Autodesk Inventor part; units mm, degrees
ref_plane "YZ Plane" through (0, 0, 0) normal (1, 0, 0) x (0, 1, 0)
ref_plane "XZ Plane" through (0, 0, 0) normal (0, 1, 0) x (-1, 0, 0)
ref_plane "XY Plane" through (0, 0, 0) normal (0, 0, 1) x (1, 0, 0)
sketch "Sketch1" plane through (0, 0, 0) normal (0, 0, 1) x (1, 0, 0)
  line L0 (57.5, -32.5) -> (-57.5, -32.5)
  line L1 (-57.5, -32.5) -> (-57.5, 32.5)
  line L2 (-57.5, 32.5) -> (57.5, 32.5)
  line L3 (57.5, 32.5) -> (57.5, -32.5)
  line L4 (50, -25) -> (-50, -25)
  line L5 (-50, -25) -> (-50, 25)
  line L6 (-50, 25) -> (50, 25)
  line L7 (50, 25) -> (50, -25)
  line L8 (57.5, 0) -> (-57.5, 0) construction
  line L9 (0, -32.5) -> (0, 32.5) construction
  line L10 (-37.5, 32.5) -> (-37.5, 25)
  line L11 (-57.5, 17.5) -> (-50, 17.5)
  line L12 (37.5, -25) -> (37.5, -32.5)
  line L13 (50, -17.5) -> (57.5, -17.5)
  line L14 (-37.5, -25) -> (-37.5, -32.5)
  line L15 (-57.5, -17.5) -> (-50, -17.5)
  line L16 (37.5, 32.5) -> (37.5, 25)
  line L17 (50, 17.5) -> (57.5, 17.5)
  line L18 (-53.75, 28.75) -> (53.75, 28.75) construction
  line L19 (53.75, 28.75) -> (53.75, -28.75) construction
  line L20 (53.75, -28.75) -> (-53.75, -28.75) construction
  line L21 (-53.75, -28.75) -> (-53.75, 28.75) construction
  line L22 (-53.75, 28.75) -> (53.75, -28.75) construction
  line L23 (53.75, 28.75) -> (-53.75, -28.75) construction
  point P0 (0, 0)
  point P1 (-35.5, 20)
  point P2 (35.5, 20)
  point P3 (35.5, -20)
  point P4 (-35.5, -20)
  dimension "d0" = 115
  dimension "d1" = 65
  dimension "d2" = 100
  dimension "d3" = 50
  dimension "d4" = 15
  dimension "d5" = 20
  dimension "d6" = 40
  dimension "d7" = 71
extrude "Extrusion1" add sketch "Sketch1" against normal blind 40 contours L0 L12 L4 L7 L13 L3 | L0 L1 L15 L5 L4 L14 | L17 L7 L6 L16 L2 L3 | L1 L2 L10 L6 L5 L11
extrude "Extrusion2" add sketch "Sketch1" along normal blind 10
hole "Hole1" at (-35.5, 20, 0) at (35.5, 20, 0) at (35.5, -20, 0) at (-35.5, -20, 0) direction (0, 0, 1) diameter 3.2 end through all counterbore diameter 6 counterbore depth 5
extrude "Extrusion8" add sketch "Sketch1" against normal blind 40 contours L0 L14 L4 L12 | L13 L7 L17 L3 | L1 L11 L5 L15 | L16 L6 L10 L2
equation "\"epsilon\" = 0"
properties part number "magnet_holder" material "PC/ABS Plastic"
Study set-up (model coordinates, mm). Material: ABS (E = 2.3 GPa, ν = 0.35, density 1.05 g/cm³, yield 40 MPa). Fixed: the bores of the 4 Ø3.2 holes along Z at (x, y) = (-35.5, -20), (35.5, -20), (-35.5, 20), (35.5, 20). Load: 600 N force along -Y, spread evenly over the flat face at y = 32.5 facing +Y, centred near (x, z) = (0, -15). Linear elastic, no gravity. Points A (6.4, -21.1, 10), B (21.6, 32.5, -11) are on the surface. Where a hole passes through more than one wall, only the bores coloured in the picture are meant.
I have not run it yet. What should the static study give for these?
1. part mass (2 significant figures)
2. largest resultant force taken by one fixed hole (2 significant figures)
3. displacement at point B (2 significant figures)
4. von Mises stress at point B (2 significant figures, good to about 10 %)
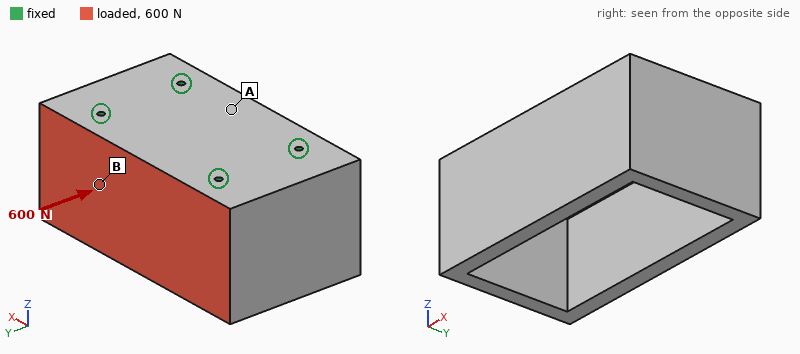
180 g
220 N
0.13 mm
2.1 MPa
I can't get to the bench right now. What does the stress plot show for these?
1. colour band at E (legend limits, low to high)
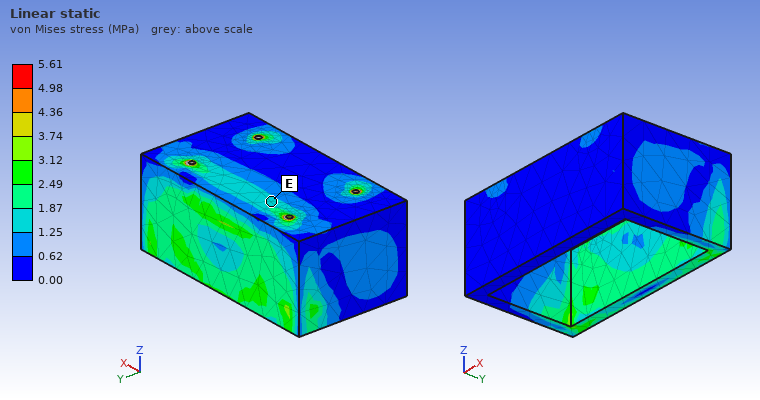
1.25 to 1.87 MPa
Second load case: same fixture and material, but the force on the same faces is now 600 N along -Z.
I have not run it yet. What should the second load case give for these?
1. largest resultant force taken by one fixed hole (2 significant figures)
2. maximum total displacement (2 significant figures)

380 N
0.20 mm
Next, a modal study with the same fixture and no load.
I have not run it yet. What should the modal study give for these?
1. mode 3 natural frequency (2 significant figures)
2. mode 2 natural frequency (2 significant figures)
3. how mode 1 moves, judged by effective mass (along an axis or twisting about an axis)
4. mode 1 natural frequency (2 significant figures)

1300 Hz
1200 Hz
along Y
1100 Hz
